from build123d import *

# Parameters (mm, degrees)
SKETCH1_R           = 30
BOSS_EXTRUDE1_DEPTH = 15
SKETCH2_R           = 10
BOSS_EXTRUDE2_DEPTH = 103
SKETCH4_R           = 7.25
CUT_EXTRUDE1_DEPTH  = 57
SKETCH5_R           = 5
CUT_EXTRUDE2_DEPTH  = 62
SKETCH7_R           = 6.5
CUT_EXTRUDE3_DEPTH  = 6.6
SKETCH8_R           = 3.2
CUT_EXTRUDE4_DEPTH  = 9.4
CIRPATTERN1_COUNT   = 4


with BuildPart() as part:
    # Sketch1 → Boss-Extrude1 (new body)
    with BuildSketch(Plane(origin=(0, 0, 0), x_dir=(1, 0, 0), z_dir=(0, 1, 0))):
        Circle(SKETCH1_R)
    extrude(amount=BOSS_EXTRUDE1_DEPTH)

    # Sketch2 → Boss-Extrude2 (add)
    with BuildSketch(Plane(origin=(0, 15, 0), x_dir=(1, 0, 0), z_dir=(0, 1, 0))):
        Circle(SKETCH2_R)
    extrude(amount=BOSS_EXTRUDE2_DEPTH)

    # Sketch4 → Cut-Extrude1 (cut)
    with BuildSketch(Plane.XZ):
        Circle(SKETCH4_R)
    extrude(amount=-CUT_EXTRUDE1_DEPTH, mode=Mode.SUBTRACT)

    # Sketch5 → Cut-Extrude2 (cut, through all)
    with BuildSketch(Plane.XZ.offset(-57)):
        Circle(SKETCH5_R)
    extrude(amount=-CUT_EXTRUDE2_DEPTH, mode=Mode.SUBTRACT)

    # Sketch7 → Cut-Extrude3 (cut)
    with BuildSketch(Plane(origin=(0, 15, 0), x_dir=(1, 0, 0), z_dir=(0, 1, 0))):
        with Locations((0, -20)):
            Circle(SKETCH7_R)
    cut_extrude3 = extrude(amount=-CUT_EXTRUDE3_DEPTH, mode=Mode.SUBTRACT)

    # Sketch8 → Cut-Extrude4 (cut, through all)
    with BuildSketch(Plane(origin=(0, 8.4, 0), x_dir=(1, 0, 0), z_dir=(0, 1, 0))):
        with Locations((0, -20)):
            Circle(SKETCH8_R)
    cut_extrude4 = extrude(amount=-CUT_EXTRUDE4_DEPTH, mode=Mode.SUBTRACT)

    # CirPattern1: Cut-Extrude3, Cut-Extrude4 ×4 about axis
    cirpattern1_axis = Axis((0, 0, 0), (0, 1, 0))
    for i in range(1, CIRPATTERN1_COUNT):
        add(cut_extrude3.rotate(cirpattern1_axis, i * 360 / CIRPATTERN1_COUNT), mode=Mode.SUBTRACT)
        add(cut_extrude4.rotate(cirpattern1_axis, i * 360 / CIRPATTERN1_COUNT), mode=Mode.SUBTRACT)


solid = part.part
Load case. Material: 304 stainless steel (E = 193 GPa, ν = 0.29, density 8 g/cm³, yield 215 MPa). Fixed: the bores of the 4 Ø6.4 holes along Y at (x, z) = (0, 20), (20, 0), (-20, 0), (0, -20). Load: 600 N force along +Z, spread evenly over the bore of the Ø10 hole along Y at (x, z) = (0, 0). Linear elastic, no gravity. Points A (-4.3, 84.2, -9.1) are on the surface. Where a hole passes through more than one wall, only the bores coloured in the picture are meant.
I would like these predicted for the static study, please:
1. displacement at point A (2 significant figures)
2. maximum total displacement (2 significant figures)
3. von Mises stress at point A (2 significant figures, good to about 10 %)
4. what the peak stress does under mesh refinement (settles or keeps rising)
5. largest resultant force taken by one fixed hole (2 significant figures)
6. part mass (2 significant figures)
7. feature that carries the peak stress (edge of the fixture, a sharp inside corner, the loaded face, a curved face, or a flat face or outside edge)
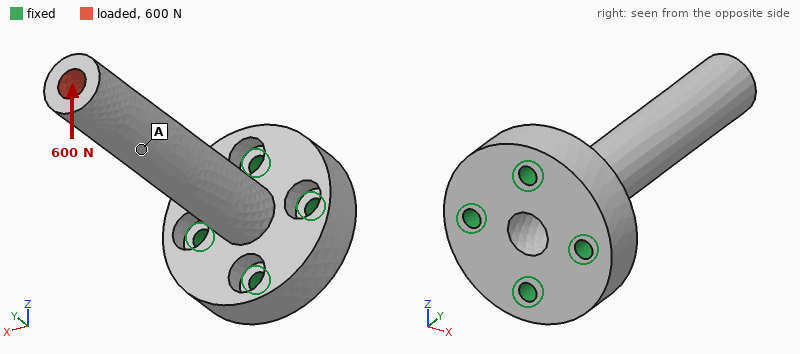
0.086 mm
0.14 mm
7.0 MPa
keeps rising
1.4 kN
450 g
a sharp inside corner
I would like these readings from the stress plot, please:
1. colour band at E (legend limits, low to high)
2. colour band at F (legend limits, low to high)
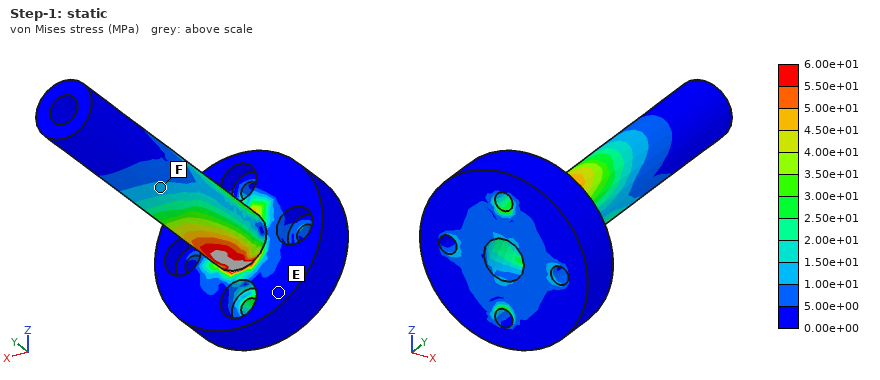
0.00e+00 to 5.00e+00 MPa
1.00e+01 to 1.50e+01 MPa
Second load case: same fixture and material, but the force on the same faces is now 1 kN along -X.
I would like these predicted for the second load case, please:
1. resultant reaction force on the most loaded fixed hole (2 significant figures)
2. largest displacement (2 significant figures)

2.3 kN
0.24 mm
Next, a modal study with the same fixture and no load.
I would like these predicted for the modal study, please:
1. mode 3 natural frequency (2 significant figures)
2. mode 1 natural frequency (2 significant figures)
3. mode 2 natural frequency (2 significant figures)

6700 Hz
1100 Hz
1100 Hz
